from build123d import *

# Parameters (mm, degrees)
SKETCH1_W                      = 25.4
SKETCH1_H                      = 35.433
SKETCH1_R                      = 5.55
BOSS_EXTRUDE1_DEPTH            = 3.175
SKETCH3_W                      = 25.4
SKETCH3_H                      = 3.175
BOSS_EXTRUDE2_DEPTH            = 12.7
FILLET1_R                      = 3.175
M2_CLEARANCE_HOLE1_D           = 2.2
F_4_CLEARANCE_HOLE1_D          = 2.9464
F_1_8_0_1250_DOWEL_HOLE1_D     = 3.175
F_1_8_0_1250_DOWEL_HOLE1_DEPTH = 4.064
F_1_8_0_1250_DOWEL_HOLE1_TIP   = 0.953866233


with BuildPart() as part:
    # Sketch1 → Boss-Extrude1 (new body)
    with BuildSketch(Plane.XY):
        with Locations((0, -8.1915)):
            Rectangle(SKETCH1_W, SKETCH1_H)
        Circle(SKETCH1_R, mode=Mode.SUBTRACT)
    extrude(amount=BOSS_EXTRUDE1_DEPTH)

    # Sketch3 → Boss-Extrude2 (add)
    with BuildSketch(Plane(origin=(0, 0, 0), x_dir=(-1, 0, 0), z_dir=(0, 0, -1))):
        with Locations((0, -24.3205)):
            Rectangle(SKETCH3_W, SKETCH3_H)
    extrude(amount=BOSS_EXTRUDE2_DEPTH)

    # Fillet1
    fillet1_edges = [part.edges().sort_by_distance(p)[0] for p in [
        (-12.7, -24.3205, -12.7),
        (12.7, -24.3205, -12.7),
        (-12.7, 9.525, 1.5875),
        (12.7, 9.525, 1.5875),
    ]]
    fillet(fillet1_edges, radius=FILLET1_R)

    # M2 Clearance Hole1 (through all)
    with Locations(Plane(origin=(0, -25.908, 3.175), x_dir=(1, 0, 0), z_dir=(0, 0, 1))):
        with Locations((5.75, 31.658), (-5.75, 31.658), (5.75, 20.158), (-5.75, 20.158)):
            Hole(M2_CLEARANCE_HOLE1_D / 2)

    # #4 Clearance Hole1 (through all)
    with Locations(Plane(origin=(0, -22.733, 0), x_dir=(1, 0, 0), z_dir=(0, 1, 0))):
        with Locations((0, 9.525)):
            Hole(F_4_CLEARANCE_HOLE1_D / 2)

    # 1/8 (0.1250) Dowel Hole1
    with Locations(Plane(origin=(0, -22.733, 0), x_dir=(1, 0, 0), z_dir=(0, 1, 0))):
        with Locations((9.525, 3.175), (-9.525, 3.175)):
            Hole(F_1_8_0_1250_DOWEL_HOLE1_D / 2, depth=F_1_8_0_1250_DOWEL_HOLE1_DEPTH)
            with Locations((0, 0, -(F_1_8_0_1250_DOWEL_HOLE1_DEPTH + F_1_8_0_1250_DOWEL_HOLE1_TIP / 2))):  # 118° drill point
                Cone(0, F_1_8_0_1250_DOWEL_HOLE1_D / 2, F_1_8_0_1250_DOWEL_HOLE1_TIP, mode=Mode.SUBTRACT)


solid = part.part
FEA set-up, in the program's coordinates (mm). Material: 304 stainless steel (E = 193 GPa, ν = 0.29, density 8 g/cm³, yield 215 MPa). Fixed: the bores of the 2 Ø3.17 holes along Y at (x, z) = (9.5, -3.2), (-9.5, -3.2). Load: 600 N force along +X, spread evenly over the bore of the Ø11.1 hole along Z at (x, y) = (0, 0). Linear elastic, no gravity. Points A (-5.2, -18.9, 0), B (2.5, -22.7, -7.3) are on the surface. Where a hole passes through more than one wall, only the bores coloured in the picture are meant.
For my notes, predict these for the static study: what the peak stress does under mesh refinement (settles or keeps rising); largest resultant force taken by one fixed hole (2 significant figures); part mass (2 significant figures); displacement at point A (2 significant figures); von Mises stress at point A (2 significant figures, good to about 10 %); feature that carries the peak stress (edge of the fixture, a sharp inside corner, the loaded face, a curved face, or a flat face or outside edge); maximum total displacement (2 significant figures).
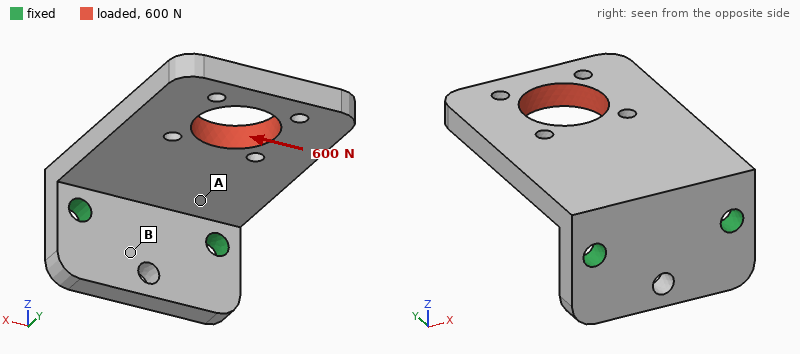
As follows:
keeps rising
810 N
27 g
4.3 µm
40 MPa
edge of the fixture
26 µm
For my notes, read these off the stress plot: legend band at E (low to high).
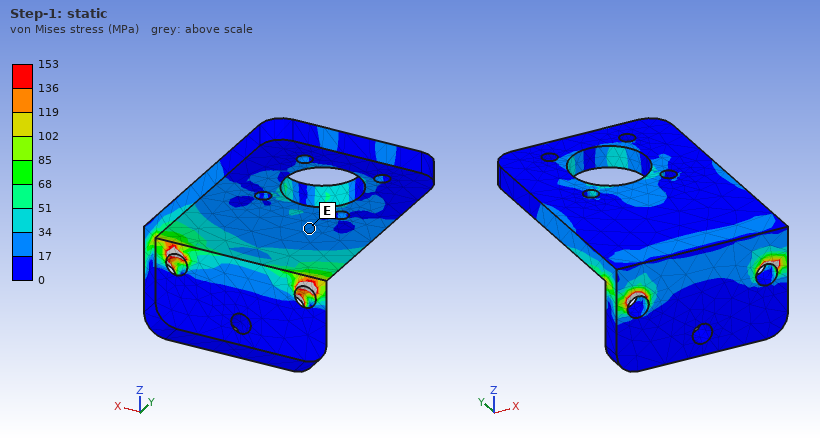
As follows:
17 to 34 MPa
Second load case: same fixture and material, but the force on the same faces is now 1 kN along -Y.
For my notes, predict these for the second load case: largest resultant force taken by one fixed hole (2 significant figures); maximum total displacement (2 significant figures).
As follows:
500 N
31 µm
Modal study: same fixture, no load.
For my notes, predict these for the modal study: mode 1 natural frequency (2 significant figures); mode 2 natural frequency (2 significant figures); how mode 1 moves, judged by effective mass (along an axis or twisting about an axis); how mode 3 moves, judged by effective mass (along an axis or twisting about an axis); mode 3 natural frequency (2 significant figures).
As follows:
2100 Hz
5800 Hz
along Z
along X
9000 Hz
